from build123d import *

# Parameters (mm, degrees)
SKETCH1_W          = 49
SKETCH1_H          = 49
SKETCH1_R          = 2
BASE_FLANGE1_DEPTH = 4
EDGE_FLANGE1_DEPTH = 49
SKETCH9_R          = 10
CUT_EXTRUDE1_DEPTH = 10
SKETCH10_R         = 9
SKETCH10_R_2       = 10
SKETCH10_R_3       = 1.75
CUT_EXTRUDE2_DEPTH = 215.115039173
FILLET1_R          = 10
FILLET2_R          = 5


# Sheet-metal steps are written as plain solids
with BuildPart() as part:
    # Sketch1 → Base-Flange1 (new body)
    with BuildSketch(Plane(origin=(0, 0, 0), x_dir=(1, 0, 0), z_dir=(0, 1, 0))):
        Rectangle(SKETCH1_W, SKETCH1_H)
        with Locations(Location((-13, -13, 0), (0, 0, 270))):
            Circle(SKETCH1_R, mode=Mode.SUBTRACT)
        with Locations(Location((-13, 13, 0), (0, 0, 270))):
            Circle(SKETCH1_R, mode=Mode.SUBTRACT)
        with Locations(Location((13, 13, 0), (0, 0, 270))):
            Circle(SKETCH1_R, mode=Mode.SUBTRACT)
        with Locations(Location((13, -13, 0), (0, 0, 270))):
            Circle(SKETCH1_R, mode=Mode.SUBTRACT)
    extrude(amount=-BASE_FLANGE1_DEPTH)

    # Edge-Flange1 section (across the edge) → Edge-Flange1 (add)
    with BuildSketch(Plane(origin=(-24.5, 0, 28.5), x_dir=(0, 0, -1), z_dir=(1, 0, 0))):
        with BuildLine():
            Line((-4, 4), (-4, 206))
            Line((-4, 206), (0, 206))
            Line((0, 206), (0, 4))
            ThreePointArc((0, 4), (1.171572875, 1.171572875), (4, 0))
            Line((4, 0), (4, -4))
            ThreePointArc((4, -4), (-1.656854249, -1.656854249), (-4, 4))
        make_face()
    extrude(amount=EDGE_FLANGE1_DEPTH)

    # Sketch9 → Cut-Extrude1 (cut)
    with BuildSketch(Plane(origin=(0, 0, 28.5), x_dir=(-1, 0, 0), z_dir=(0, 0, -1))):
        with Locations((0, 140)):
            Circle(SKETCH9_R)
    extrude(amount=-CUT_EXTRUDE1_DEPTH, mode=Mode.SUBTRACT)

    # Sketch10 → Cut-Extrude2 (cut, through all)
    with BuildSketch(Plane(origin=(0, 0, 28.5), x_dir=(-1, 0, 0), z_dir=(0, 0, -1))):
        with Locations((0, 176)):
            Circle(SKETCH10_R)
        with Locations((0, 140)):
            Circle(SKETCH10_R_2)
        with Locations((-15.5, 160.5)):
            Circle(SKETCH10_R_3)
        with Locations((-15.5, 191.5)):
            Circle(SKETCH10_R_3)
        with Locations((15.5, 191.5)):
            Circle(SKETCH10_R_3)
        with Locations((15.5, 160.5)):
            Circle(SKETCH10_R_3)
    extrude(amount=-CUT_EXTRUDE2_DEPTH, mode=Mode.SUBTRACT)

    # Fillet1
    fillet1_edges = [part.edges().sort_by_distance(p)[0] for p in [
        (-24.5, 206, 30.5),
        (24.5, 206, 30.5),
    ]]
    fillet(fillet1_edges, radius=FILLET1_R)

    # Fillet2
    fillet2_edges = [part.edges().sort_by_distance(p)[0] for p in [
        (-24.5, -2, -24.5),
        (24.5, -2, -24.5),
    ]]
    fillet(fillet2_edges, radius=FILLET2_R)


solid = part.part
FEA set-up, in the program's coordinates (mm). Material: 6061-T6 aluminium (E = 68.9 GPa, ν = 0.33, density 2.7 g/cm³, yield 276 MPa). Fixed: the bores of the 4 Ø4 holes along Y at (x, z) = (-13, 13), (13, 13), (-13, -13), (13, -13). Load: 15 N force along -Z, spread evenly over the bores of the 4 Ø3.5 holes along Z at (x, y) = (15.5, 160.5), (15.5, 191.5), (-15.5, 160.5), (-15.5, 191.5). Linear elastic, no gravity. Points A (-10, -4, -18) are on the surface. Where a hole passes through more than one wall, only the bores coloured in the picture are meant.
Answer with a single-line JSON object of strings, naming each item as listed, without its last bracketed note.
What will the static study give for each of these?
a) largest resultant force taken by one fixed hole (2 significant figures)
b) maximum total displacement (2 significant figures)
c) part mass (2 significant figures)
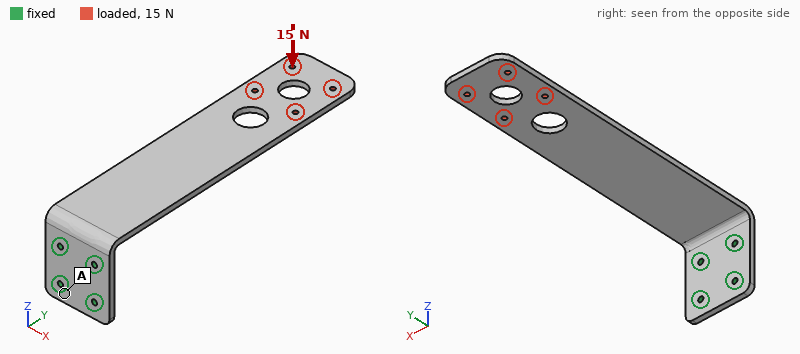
{"largest resultant force taken by one fixed hole": "22 N", "maximum total displacement": "2.4 mm", "part mass": "130 g"}
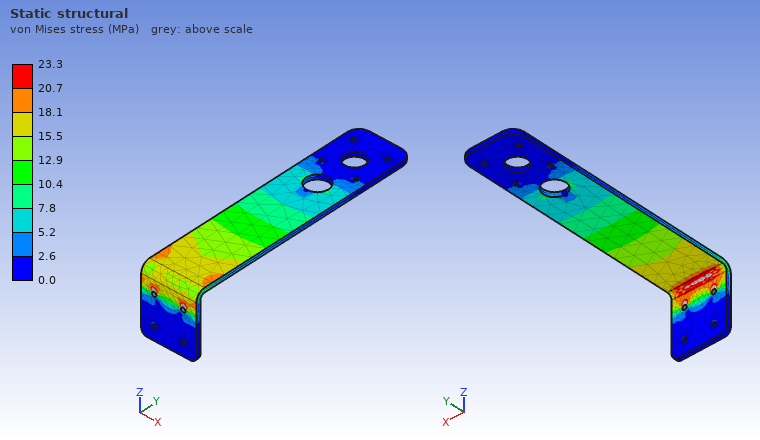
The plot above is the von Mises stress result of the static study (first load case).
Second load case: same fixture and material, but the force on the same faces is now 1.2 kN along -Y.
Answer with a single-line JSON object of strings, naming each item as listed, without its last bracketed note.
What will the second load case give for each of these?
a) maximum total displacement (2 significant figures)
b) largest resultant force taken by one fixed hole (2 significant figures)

{"maximum total displacement": "2.2 mm", "largest resultant force taken by one fixed hole": "710 N"}
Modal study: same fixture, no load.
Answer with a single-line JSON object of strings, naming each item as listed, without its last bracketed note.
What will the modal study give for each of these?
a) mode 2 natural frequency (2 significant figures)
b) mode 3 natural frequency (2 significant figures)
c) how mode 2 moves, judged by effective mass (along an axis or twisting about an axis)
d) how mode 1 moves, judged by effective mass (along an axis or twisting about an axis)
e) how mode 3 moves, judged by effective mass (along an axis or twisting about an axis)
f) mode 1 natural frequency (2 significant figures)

{"mode 2 natural frequency": "280 Hz", "mode 3 natural frequency": "420 Hz", "how mode 2 moves, judged by effective mass": "along X", "how mode 1 moves, judged by effective mass": "along Z", "how mode 3 moves, judged by effective mass": "along Z", "mode 1 natural frequency": "72 Hz"}
